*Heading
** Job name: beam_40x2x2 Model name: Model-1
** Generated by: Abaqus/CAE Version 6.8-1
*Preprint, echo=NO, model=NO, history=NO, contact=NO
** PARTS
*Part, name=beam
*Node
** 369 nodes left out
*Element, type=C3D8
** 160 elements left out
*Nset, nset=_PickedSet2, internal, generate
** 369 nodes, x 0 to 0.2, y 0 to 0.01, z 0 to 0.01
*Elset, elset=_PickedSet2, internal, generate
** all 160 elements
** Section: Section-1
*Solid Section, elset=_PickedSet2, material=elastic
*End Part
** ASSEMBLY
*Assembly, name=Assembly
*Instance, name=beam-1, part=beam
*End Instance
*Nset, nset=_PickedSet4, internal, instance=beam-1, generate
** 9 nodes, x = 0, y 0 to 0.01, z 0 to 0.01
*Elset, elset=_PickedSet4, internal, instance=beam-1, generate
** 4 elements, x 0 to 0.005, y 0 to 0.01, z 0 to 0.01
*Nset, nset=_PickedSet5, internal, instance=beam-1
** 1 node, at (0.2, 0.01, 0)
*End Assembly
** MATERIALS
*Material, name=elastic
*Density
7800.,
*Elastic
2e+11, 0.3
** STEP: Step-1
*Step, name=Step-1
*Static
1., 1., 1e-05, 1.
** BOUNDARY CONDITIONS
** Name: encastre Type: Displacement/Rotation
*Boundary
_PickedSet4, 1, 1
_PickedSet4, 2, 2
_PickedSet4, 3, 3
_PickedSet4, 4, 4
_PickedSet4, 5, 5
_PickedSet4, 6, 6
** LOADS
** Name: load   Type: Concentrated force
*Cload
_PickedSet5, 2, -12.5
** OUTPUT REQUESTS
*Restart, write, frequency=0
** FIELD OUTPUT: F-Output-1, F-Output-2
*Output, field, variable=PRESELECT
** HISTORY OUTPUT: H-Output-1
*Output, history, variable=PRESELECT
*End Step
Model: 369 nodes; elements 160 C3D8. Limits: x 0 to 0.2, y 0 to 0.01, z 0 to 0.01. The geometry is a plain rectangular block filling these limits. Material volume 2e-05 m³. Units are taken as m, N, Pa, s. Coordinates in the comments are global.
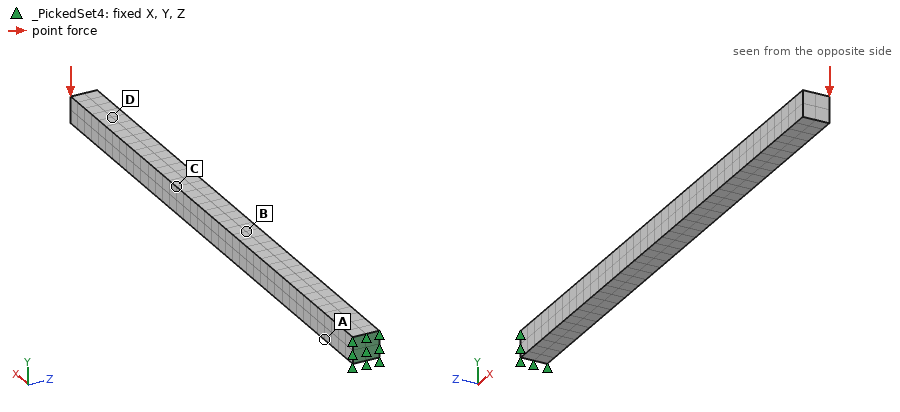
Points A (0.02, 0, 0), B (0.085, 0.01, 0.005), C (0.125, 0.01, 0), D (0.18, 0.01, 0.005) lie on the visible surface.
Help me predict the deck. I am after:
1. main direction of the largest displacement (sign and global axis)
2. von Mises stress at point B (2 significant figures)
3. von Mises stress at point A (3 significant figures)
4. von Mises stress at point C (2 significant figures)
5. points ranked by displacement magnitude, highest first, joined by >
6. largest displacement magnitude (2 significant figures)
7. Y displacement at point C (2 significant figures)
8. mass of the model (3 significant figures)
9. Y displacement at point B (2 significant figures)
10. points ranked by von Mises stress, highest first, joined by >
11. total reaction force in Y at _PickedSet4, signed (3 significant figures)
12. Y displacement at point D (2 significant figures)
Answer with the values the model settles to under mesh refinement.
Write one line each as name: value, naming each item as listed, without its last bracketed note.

main direction of the largest displacement: -Y
von Mises stress at point B: 8.6e+06 Pa
von Mises stress at point A: 1.35e+07 Pa
von Mises stress at point C: 5.6e+06 Pa
points ranked by displacement magnitude, highest first, joined by >: D > C > B > A
largest displacement magnitude: 2.0e-04 m
Y displacement at point C: -9.3e-05 m
mass of the model: 0.156 kg
Y displacement at point B: -4.6e-05 m
points ranked by von Mises stress, highest first, joined by >: A > B > C > D
total reaction force in Y at _PickedSet4, signed: 12.5 N
Y displacement at point D: -1.7e-04 m
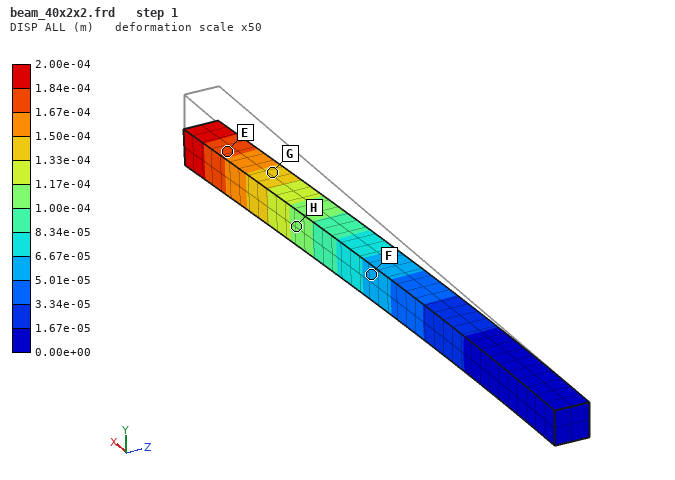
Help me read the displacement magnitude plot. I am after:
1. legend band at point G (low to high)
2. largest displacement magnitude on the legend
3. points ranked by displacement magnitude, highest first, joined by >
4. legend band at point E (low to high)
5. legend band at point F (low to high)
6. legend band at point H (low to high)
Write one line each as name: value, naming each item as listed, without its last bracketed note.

legend band at point G: 1.33e-04 to 1.50e-04 m
largest displacement magnitude on the legend: 2.00e-04 m
points ranked by displacement magnitude, highest first, joined by >: E > G > H > F
legend band at point E: 1.67e-04 to 1.84e-04 m
legend band at point F: 5.01e-05 to 6.67e-05 m
legend band at point H: 1.00e-04 to 1.17e-04 m
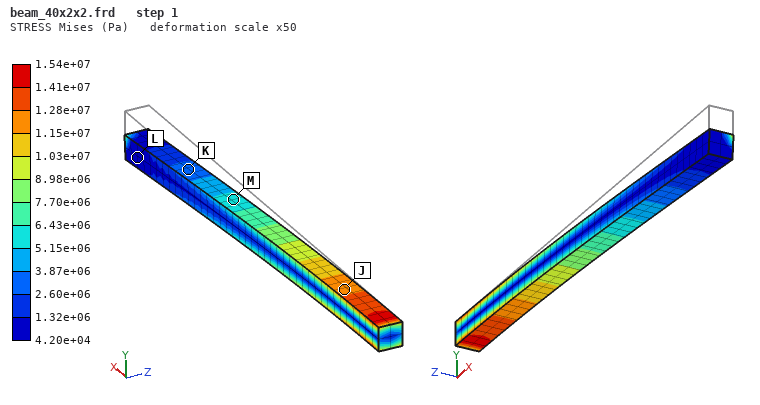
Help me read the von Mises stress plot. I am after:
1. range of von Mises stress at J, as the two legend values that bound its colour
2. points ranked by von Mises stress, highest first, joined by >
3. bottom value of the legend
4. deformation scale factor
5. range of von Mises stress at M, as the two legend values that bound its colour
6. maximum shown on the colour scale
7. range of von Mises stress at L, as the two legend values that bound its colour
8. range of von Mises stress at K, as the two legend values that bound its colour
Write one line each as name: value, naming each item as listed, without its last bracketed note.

range of von Mises stress at J, as the two legend values that bound its colour: 1.15e+07 to 1.28e+07 Pa
points ranked by von Mises stress, highest first, joined by >: J > M > K > L
bottom value of the legend: 4.20e+04 Pa
deformation scale factor: 50
range of von Mises stress at M, as the two legend values that bound its colour: 5.15e+06 to 6.43e+06 Pa
maximum shown on the colour scale: 1.54e+07 Pa
range of von Mises stress at L, as the two legend values that bound its colour: 4.20e+04 to 1.32e+06 Pa
range of von Mises stress at K, as the two legend values that bound its colour: 2.60e+06 to 3.87e+06 Pa
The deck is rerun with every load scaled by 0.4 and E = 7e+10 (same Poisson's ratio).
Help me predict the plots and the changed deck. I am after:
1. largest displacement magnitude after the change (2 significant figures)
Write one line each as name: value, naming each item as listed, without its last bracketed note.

largest displacement magnitude after the change: 2.3e-04 m
